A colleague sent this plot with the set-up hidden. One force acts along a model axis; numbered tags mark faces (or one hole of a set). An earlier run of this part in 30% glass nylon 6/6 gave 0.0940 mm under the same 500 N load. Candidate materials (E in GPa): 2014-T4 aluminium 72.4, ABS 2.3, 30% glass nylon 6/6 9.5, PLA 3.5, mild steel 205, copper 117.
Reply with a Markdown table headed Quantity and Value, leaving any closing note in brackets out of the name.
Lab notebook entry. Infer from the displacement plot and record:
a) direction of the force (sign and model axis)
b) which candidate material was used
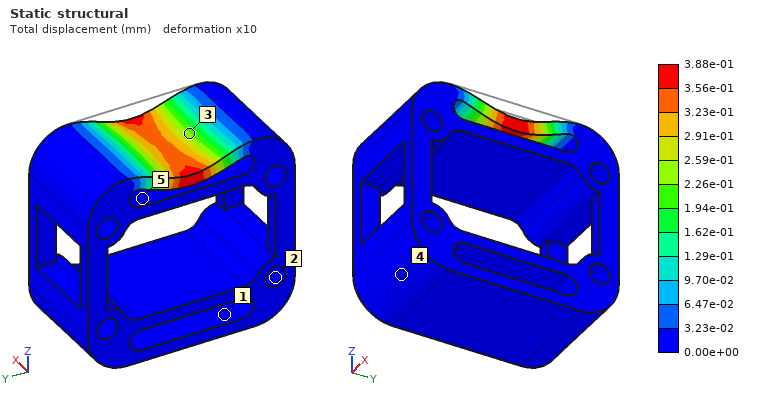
| Quantity | Value |
|---|---|
| direction of the force | -Z |
| which candidate material was used | ABS |
